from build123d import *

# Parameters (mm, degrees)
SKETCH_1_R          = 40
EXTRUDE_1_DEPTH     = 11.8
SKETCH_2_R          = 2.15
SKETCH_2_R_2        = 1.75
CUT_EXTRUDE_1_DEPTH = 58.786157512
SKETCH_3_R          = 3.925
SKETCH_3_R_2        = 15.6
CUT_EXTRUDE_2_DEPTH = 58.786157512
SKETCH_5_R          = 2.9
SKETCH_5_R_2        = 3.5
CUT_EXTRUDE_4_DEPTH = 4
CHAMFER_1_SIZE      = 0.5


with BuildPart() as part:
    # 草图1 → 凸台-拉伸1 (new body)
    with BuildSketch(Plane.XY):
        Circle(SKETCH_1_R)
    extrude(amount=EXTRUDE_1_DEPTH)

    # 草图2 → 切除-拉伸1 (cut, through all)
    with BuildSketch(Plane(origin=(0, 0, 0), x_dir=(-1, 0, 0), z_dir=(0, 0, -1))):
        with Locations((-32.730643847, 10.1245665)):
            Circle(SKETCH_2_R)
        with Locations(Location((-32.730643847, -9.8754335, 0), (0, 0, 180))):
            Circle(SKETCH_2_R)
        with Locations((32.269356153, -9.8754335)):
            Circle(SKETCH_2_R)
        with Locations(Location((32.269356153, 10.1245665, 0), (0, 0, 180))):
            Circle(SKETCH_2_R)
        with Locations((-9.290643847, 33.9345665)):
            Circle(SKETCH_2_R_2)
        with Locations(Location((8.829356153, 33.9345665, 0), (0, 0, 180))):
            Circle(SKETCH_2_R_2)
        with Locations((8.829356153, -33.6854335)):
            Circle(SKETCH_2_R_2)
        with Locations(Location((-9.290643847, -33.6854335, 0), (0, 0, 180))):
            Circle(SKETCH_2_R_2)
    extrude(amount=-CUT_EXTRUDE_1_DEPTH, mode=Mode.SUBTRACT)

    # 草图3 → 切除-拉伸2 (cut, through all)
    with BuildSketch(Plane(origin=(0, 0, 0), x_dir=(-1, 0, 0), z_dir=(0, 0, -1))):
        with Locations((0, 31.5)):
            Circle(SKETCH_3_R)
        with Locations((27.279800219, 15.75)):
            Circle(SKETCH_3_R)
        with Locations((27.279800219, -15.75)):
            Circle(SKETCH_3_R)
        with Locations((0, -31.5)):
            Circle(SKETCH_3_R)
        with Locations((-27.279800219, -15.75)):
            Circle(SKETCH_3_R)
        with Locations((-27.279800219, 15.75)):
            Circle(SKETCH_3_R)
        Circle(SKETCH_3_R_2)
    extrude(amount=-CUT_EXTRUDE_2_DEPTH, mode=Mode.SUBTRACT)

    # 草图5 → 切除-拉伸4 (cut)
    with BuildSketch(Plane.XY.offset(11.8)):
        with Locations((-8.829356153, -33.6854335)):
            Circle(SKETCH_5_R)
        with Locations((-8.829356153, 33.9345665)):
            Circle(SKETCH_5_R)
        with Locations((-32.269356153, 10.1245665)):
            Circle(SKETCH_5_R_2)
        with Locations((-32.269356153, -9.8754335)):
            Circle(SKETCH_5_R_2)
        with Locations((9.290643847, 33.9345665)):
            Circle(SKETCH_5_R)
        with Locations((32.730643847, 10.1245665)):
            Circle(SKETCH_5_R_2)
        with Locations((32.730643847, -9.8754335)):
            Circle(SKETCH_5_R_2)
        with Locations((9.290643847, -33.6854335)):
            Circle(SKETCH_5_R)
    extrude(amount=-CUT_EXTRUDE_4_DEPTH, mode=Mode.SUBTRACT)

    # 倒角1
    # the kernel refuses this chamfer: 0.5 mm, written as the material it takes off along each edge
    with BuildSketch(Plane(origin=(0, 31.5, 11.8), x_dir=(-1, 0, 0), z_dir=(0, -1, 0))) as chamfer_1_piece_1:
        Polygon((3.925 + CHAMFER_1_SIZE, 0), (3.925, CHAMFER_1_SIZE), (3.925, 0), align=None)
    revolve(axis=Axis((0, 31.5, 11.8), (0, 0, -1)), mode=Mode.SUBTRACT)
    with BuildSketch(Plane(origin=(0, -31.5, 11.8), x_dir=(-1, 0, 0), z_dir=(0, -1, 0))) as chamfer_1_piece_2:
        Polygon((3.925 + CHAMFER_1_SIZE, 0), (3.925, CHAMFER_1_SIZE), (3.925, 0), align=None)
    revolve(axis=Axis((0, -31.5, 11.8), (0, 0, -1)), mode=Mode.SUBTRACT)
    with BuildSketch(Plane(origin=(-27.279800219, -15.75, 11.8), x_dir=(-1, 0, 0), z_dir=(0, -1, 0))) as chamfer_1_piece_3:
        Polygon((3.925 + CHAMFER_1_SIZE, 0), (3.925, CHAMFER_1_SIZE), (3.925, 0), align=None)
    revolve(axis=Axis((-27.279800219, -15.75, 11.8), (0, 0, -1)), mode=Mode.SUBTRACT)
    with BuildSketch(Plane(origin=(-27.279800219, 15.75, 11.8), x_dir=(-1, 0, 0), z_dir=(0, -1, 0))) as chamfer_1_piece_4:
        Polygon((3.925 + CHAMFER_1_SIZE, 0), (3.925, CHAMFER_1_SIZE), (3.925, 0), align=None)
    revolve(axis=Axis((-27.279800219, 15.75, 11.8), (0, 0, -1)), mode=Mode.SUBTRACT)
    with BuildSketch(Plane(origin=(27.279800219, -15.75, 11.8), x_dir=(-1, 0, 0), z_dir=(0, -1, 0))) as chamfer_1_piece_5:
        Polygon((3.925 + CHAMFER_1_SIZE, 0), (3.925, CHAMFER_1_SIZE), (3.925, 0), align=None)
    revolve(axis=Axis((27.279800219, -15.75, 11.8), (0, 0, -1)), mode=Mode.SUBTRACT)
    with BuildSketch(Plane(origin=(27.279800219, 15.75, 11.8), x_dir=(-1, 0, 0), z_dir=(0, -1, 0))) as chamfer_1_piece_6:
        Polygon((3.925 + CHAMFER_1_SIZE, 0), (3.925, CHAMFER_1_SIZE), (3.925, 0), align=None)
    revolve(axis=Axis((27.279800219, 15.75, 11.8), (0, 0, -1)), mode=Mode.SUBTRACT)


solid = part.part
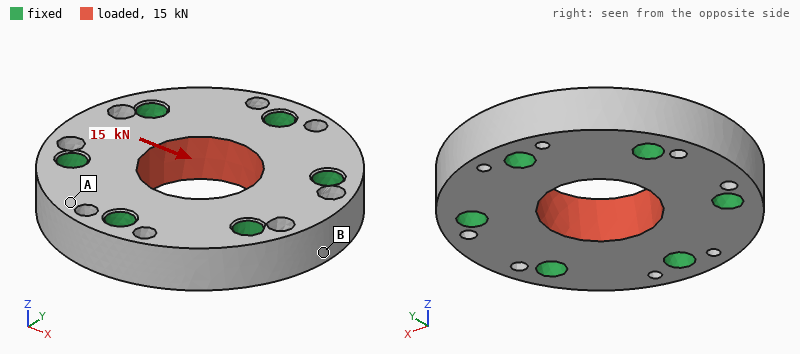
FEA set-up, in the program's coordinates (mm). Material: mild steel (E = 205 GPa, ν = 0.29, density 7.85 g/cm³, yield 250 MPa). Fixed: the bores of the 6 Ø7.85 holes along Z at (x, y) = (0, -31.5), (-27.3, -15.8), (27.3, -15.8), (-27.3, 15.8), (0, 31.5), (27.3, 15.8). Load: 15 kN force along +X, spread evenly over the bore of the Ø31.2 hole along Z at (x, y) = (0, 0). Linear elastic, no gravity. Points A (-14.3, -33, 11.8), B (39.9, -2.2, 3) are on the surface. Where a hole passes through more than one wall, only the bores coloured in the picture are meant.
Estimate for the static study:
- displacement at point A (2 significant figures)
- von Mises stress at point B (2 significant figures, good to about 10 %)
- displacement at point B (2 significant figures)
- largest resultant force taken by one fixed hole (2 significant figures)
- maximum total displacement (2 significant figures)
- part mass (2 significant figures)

0.32 µm
6.0 MPa
0.74 µm
3.2 kN
1.5 µm
350 g
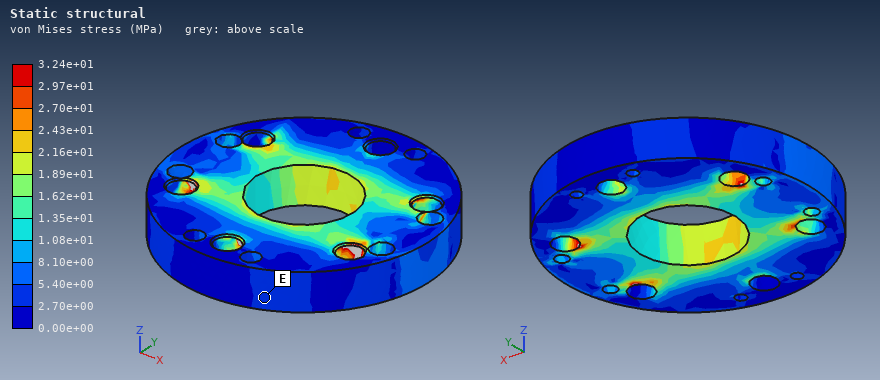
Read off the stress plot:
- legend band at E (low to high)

2.70e+00 to 5.40e+00 MPa
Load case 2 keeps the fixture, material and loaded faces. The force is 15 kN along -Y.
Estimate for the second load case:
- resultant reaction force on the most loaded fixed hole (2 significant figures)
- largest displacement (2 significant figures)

3.5 kN
1.4 µm
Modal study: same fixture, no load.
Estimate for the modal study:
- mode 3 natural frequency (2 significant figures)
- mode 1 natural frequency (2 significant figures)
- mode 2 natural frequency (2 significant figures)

33 kHz
32 kHz
32 kHz
